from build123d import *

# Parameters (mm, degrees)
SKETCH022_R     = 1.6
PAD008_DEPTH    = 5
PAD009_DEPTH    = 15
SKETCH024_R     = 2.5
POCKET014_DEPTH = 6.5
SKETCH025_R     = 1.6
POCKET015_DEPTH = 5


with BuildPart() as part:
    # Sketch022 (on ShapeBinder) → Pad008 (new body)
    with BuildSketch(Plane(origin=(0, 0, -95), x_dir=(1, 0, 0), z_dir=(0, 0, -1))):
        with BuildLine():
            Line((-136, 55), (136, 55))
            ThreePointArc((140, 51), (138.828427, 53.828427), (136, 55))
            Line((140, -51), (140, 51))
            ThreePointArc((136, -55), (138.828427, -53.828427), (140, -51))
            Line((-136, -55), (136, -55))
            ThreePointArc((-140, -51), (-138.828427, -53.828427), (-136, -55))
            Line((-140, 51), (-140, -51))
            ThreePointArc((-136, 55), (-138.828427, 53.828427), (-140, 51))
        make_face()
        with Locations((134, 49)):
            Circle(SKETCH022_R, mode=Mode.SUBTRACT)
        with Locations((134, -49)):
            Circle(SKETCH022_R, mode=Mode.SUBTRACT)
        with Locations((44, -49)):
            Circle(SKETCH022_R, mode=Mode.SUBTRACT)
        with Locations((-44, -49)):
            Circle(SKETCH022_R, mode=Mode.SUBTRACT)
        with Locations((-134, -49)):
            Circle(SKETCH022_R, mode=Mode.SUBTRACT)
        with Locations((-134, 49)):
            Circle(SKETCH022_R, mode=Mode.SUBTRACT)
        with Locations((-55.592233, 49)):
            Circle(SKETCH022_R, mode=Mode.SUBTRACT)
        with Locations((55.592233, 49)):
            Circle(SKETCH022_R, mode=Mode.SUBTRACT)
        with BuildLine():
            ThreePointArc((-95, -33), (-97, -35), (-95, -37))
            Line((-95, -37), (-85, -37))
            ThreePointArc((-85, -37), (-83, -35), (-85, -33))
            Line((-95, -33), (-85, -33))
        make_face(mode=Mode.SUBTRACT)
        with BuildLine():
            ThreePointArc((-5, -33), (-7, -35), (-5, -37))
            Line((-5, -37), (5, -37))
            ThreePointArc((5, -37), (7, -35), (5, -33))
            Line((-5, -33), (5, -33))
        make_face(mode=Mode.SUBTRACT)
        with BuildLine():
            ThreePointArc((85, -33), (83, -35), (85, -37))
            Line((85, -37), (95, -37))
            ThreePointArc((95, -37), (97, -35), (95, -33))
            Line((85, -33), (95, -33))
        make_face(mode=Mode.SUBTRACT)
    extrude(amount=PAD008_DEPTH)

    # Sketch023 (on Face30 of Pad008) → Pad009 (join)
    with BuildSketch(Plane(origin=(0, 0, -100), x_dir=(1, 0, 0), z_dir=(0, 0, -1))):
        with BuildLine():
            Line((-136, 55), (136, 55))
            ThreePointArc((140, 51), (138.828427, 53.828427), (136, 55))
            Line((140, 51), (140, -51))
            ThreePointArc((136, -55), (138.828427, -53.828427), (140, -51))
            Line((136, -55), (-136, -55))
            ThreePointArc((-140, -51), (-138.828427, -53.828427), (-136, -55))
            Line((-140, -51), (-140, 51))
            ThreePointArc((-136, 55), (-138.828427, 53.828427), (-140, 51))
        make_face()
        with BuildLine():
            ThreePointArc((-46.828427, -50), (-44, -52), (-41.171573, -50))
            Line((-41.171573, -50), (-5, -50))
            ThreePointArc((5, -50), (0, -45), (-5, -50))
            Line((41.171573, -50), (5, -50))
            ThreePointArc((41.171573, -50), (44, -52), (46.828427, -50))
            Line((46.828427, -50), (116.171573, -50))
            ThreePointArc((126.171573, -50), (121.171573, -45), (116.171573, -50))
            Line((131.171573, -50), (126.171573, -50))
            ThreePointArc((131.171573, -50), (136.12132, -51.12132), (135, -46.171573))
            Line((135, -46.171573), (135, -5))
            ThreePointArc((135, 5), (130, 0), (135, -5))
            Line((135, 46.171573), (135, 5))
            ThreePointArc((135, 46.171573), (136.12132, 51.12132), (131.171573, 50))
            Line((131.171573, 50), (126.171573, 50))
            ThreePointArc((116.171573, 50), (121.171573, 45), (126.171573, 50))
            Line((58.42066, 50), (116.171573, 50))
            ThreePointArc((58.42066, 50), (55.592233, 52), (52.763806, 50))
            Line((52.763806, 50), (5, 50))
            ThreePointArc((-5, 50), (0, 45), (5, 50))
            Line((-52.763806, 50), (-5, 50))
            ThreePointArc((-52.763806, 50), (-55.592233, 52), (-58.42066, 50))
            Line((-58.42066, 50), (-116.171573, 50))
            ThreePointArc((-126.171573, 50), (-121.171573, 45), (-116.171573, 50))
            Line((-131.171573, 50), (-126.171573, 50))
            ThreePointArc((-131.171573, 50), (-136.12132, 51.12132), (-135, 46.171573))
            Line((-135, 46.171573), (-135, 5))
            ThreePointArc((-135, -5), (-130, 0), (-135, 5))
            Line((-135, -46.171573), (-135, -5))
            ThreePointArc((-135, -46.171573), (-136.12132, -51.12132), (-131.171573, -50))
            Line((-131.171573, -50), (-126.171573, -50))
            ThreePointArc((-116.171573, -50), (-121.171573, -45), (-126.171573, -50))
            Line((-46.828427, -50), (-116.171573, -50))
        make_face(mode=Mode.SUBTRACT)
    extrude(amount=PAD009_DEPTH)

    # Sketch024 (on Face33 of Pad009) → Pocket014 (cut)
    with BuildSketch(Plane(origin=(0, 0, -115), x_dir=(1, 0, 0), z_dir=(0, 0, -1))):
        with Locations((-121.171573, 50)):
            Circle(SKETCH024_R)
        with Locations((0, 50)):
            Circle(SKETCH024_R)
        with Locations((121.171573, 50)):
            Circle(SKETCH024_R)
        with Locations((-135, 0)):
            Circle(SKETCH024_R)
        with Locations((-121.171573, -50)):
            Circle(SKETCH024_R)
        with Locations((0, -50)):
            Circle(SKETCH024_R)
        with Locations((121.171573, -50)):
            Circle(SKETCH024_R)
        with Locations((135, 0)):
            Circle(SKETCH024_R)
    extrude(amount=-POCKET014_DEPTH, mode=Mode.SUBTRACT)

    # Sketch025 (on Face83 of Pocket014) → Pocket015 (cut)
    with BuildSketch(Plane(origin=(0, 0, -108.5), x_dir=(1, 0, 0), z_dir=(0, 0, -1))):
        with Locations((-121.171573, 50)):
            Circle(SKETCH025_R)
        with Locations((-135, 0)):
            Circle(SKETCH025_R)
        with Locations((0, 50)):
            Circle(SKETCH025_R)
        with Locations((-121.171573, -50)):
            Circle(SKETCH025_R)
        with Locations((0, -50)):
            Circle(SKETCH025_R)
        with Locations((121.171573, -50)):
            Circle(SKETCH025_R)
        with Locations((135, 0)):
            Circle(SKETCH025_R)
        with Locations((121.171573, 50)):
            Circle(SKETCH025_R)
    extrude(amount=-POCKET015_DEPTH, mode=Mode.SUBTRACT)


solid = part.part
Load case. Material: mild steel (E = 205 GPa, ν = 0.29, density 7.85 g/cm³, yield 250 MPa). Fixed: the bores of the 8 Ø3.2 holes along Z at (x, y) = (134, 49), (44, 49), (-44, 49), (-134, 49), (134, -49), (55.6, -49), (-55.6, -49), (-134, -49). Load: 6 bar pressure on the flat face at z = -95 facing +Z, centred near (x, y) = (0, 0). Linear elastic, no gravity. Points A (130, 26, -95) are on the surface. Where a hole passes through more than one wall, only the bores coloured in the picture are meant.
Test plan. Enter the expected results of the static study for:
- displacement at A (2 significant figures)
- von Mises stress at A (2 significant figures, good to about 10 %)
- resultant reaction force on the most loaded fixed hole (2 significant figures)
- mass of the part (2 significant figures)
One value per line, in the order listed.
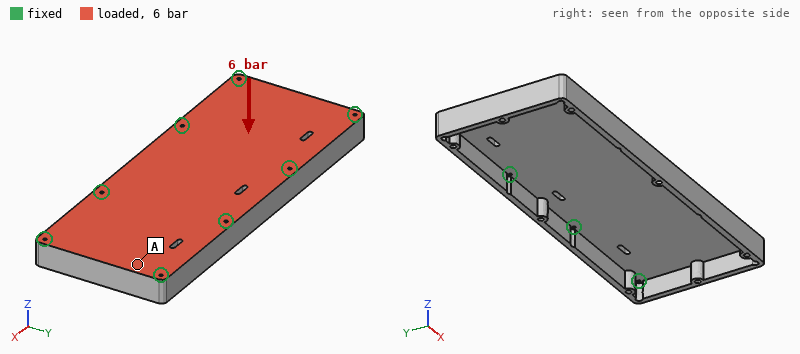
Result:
0.024 mm
30 MPa
3.4 kN
1.7 kg
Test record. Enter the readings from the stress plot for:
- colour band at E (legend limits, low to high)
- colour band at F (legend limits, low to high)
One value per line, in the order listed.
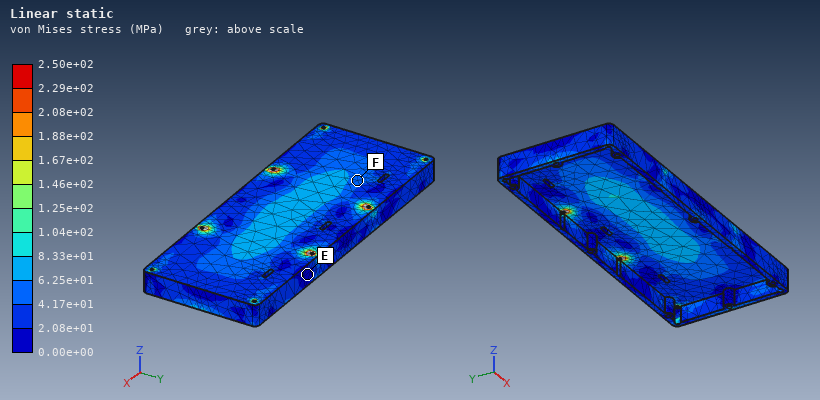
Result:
0.00e+00 to 2.08e+01 MPa
4.17e+01 to 6.25e+01 MPa
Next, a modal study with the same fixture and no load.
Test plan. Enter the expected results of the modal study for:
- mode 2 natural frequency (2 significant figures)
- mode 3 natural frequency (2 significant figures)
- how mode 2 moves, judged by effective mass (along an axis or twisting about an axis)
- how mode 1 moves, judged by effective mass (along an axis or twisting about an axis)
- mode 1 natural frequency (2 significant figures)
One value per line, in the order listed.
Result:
2400 Hz
2700 Hz
twisting about Y
along Z
1900 Hz
